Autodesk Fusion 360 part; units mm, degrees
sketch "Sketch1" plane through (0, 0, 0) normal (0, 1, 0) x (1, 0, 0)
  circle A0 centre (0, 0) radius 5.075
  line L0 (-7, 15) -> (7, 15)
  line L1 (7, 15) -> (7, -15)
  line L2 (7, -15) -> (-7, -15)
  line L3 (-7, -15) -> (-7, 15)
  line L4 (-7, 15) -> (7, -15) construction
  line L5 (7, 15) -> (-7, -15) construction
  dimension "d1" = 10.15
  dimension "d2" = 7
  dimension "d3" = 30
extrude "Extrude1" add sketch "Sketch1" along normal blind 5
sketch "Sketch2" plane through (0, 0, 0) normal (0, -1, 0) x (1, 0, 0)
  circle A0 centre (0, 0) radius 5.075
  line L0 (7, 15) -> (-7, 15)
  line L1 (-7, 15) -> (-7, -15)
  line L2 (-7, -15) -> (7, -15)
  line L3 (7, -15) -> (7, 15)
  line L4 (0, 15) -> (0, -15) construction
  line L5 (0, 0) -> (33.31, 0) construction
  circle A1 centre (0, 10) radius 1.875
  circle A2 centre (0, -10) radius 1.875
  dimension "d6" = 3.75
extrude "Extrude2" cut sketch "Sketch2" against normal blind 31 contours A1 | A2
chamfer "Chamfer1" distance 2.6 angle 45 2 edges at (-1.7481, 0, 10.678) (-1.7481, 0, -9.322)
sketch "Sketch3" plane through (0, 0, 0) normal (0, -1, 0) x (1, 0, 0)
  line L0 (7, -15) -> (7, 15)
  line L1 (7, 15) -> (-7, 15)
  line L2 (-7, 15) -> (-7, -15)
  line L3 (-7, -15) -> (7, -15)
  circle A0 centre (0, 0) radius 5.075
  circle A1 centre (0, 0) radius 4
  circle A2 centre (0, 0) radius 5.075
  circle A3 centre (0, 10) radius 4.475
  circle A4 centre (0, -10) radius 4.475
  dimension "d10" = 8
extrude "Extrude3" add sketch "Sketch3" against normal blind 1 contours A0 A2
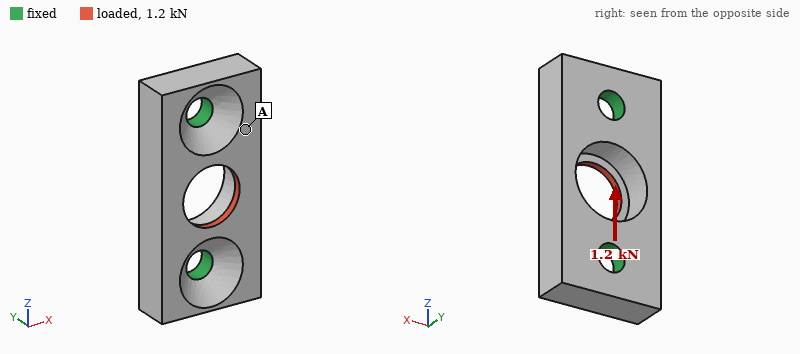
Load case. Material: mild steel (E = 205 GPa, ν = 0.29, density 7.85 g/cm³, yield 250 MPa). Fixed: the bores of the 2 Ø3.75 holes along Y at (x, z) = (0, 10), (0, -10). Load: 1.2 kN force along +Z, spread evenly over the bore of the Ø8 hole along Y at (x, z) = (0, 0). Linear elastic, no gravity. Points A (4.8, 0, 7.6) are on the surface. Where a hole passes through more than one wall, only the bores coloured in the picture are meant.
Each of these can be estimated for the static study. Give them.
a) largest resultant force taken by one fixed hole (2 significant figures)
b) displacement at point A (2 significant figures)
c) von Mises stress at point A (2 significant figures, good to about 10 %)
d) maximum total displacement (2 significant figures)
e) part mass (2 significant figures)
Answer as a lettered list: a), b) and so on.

a) 620 N
b) 0.99 µm
c) 15 MPa
d) 2.7 µm
e) 12 g
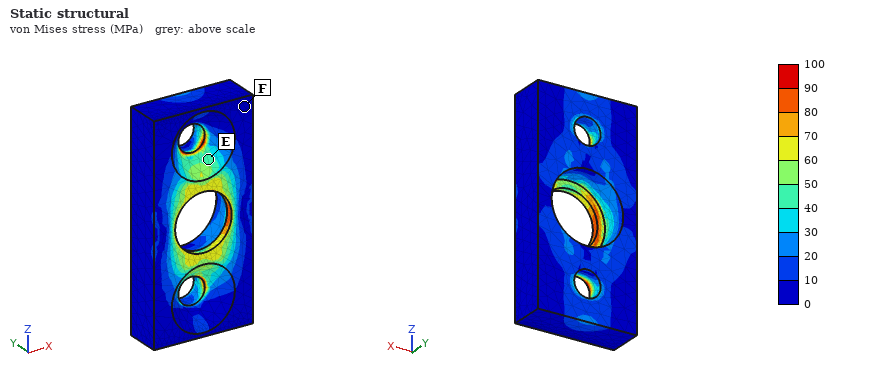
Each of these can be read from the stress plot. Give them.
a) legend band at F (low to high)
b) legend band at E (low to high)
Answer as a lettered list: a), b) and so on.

a) 0 to 10 MPa
b) 40 to 50 MPa
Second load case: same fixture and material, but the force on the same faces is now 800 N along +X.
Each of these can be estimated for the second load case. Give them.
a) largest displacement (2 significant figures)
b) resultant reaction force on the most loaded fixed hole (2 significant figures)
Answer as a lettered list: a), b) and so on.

a) 4.7 µm
b) 400 N
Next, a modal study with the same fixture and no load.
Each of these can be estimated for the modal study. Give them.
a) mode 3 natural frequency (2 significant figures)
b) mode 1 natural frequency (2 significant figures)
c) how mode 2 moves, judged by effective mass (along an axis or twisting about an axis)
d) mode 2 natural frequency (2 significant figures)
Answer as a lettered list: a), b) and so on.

a) 42 kHz
b) 30 kHz
c) along Y
d) 39 kHz
